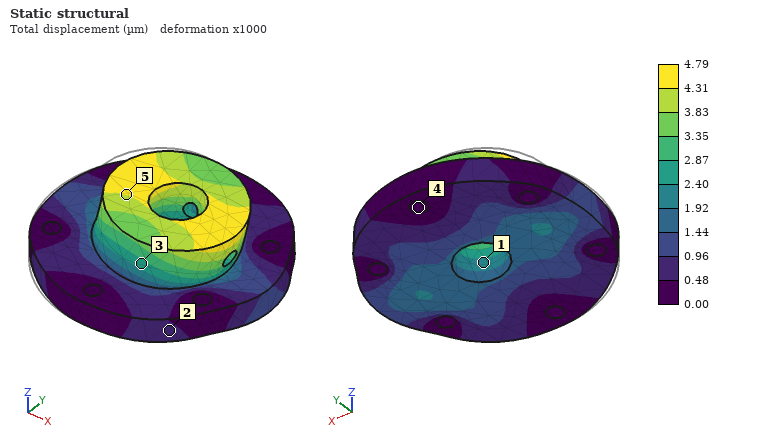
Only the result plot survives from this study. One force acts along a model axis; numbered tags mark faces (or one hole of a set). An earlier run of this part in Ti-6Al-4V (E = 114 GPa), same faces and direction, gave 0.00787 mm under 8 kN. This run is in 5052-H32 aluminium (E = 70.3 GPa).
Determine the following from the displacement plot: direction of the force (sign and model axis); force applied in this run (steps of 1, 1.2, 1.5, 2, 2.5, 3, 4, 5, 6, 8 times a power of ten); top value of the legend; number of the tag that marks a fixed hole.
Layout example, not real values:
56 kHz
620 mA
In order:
+X
3 kN
4.79 µm
4
